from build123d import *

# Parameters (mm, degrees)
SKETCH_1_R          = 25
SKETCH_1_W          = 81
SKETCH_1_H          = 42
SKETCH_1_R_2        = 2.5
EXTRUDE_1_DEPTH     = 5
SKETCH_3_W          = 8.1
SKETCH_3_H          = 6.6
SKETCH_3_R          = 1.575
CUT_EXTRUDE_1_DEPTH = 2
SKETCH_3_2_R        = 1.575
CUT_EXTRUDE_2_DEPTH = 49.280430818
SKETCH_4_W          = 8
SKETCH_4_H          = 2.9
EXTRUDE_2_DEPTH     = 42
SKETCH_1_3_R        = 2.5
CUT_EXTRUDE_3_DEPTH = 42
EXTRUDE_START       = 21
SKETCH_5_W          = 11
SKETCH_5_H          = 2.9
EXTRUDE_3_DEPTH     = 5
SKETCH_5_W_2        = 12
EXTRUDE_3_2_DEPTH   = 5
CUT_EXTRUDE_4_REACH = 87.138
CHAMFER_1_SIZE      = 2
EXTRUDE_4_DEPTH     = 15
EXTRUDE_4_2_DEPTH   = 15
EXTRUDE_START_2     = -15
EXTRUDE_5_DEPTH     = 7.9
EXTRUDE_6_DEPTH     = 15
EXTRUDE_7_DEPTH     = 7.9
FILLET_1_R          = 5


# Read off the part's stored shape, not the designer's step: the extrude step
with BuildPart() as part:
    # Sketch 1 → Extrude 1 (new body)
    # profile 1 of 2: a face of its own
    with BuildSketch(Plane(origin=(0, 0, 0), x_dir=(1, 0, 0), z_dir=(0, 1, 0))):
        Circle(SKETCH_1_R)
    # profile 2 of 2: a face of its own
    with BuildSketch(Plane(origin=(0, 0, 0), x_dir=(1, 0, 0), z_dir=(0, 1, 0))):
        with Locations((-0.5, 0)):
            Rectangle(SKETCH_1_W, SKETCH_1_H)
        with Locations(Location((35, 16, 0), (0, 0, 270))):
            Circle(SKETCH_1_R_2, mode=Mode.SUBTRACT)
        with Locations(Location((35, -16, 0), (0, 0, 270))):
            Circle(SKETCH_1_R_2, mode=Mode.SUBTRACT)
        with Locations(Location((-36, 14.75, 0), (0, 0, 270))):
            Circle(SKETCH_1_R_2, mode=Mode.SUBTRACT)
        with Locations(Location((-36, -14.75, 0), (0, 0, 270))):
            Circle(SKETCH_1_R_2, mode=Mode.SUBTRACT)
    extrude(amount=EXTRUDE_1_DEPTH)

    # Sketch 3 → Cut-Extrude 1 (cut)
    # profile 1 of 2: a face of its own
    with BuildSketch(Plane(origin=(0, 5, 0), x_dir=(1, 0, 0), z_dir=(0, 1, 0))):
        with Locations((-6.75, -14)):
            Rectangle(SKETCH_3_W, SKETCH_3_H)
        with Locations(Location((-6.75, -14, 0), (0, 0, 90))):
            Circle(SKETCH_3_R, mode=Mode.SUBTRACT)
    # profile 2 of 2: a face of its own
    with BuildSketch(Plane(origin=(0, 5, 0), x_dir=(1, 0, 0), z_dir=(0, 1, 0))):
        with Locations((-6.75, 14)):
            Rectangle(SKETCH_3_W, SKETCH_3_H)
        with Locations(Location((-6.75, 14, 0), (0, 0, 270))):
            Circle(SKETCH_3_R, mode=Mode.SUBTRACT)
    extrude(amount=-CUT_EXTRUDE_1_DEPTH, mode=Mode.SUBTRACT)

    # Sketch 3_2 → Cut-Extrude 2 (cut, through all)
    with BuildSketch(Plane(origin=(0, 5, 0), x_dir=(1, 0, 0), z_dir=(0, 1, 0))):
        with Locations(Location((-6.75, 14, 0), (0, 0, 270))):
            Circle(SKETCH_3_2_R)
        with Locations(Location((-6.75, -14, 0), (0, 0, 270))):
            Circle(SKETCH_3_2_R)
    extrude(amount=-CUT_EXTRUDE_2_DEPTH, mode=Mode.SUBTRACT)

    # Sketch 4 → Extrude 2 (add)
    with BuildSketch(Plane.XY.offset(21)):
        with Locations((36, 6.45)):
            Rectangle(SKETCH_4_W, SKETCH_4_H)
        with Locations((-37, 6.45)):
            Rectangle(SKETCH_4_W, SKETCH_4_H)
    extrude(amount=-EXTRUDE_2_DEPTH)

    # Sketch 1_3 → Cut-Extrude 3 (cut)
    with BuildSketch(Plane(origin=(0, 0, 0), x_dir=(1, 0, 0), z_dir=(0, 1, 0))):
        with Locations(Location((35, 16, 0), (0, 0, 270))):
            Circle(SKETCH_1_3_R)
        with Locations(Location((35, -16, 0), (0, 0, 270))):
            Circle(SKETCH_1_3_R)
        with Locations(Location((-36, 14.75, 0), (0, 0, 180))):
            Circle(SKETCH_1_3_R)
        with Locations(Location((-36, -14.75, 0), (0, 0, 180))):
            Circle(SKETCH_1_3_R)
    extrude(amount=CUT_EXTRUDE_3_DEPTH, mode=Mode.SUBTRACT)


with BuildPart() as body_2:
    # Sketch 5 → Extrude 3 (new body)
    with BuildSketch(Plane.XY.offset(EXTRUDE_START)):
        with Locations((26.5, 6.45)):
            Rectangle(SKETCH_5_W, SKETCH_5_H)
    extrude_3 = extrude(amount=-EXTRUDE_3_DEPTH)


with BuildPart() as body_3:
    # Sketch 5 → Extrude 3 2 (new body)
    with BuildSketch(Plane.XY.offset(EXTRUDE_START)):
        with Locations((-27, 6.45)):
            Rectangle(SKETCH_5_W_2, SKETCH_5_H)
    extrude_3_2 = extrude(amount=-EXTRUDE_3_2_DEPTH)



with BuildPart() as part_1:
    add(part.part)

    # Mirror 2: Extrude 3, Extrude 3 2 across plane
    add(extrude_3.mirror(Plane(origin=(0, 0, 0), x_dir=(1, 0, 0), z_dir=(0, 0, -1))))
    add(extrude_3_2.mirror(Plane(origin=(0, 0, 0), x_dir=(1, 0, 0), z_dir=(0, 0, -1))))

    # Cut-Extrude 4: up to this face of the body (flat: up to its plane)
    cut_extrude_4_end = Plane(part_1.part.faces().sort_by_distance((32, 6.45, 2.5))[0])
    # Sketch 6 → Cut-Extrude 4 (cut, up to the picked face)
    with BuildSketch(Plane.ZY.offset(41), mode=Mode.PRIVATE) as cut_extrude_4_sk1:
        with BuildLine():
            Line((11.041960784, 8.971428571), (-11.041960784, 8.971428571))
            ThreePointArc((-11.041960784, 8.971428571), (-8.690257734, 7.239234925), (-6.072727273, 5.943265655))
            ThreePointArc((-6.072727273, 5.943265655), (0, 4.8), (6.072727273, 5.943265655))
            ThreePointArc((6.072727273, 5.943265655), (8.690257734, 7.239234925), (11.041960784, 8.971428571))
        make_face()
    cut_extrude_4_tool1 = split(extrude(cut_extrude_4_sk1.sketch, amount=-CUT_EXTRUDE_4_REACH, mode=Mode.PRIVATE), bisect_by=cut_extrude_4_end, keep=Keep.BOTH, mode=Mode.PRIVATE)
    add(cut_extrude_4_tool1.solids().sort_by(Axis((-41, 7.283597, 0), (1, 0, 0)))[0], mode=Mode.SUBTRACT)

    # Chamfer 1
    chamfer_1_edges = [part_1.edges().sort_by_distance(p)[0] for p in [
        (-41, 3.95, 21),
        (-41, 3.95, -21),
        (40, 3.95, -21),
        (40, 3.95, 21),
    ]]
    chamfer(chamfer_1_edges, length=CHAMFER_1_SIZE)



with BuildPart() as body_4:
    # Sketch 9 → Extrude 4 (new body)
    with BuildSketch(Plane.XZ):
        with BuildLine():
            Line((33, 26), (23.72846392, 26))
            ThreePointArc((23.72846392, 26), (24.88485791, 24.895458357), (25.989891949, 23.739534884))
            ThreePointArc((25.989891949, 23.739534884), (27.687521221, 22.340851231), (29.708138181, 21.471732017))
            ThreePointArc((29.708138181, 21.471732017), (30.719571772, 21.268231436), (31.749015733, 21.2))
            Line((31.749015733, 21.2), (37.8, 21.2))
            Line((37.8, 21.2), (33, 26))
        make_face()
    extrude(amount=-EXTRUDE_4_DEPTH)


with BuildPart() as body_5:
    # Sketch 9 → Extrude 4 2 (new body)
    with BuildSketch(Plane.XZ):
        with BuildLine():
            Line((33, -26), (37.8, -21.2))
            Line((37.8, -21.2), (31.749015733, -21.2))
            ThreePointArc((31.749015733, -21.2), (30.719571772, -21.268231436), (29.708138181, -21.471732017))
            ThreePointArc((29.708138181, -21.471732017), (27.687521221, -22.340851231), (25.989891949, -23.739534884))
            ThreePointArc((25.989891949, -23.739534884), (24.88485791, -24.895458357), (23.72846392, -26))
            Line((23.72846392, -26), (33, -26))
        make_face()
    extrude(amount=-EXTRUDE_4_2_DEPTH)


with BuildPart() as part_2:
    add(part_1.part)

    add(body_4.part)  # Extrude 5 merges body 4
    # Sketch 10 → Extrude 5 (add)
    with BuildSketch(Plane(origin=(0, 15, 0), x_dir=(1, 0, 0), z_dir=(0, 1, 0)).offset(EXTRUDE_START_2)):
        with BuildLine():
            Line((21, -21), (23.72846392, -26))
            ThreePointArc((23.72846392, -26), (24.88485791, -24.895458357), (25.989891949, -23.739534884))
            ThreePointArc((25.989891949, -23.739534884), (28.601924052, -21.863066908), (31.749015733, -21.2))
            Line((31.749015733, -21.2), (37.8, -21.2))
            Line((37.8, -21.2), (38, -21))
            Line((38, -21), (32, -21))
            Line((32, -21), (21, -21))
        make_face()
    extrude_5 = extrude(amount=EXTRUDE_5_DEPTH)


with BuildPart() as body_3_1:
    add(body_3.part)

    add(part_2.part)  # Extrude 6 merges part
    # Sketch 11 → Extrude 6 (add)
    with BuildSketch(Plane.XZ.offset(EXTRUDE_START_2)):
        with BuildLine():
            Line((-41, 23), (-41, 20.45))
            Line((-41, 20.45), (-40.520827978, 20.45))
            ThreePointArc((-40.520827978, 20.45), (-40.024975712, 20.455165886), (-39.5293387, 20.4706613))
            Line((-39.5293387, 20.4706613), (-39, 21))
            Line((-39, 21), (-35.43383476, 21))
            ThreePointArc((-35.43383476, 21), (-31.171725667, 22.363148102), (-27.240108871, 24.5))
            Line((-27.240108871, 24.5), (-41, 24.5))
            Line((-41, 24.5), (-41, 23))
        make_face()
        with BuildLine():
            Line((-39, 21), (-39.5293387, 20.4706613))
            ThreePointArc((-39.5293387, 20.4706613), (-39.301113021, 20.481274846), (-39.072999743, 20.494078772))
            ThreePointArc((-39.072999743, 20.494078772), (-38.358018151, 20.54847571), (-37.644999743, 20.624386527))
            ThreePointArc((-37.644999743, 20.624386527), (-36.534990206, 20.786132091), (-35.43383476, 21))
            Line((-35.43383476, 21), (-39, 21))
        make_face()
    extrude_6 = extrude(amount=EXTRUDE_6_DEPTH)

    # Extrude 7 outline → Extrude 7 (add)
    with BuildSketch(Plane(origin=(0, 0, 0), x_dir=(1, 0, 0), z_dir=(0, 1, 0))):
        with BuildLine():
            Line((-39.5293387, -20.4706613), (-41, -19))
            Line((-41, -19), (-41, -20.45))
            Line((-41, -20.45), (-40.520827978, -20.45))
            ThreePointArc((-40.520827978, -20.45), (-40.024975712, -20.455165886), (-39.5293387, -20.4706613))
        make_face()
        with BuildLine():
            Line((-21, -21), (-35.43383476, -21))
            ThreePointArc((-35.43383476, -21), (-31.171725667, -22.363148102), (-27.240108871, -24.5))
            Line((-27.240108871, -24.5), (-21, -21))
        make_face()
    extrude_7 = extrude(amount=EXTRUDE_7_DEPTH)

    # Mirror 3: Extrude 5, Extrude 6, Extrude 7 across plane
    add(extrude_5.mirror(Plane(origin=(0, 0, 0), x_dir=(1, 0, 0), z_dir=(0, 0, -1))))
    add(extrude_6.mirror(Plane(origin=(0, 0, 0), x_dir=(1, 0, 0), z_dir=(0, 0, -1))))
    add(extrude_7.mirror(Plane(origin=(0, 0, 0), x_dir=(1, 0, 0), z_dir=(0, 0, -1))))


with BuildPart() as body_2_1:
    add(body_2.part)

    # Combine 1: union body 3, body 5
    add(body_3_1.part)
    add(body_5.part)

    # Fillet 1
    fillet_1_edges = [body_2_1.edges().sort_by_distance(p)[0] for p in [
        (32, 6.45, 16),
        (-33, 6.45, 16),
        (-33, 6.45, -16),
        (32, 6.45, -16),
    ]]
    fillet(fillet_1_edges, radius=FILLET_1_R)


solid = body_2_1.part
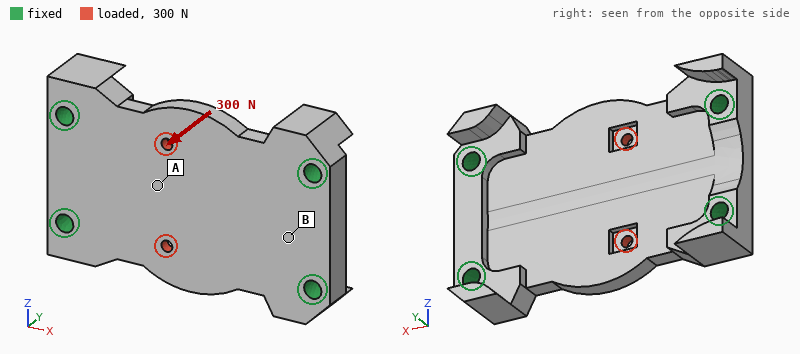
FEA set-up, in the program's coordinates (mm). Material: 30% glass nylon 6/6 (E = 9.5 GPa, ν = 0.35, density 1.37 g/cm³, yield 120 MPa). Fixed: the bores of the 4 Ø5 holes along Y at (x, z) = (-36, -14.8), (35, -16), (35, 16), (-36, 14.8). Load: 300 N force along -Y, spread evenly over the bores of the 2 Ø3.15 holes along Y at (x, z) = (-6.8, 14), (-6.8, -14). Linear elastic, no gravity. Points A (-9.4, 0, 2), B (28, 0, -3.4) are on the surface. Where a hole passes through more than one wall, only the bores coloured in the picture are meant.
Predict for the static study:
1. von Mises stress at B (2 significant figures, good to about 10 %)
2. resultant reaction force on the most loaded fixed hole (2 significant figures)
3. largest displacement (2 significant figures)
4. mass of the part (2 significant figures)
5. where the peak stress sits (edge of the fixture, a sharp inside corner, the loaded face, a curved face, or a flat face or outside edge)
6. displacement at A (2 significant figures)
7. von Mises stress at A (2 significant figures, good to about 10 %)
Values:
3.1 MPa
120 N
96 µm
31 g
the loaded face
74 µm
7.1 MPa
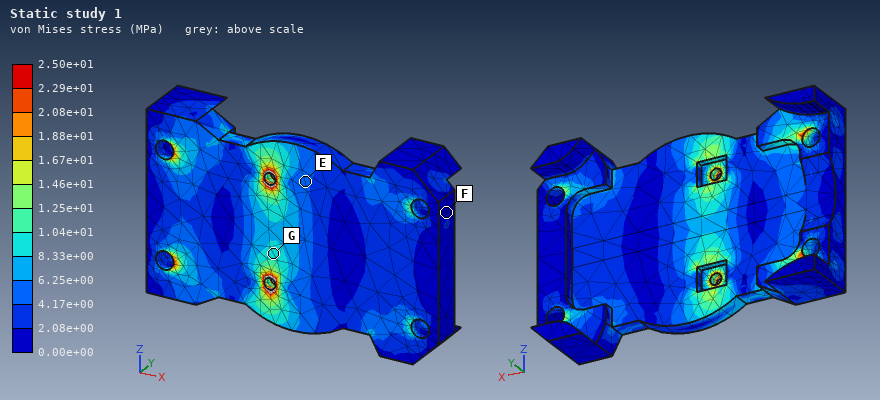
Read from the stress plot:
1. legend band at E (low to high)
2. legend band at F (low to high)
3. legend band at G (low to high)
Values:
4.17e+00 to 6.25e+00 MPa
0.00e+00 to 2.08e+00 MPa
8.33e+00 to 1.04e+01 MPa
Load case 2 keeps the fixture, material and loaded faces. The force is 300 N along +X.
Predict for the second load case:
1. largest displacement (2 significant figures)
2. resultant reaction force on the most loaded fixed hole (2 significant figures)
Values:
5.2 µm
87 N
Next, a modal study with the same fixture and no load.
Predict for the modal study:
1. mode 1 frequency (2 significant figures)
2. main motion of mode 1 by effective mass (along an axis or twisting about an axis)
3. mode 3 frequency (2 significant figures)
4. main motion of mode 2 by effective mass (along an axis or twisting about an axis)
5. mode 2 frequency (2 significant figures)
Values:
3300 Hz
along Y
7700 Hz
twisting about X
4400 Hz
